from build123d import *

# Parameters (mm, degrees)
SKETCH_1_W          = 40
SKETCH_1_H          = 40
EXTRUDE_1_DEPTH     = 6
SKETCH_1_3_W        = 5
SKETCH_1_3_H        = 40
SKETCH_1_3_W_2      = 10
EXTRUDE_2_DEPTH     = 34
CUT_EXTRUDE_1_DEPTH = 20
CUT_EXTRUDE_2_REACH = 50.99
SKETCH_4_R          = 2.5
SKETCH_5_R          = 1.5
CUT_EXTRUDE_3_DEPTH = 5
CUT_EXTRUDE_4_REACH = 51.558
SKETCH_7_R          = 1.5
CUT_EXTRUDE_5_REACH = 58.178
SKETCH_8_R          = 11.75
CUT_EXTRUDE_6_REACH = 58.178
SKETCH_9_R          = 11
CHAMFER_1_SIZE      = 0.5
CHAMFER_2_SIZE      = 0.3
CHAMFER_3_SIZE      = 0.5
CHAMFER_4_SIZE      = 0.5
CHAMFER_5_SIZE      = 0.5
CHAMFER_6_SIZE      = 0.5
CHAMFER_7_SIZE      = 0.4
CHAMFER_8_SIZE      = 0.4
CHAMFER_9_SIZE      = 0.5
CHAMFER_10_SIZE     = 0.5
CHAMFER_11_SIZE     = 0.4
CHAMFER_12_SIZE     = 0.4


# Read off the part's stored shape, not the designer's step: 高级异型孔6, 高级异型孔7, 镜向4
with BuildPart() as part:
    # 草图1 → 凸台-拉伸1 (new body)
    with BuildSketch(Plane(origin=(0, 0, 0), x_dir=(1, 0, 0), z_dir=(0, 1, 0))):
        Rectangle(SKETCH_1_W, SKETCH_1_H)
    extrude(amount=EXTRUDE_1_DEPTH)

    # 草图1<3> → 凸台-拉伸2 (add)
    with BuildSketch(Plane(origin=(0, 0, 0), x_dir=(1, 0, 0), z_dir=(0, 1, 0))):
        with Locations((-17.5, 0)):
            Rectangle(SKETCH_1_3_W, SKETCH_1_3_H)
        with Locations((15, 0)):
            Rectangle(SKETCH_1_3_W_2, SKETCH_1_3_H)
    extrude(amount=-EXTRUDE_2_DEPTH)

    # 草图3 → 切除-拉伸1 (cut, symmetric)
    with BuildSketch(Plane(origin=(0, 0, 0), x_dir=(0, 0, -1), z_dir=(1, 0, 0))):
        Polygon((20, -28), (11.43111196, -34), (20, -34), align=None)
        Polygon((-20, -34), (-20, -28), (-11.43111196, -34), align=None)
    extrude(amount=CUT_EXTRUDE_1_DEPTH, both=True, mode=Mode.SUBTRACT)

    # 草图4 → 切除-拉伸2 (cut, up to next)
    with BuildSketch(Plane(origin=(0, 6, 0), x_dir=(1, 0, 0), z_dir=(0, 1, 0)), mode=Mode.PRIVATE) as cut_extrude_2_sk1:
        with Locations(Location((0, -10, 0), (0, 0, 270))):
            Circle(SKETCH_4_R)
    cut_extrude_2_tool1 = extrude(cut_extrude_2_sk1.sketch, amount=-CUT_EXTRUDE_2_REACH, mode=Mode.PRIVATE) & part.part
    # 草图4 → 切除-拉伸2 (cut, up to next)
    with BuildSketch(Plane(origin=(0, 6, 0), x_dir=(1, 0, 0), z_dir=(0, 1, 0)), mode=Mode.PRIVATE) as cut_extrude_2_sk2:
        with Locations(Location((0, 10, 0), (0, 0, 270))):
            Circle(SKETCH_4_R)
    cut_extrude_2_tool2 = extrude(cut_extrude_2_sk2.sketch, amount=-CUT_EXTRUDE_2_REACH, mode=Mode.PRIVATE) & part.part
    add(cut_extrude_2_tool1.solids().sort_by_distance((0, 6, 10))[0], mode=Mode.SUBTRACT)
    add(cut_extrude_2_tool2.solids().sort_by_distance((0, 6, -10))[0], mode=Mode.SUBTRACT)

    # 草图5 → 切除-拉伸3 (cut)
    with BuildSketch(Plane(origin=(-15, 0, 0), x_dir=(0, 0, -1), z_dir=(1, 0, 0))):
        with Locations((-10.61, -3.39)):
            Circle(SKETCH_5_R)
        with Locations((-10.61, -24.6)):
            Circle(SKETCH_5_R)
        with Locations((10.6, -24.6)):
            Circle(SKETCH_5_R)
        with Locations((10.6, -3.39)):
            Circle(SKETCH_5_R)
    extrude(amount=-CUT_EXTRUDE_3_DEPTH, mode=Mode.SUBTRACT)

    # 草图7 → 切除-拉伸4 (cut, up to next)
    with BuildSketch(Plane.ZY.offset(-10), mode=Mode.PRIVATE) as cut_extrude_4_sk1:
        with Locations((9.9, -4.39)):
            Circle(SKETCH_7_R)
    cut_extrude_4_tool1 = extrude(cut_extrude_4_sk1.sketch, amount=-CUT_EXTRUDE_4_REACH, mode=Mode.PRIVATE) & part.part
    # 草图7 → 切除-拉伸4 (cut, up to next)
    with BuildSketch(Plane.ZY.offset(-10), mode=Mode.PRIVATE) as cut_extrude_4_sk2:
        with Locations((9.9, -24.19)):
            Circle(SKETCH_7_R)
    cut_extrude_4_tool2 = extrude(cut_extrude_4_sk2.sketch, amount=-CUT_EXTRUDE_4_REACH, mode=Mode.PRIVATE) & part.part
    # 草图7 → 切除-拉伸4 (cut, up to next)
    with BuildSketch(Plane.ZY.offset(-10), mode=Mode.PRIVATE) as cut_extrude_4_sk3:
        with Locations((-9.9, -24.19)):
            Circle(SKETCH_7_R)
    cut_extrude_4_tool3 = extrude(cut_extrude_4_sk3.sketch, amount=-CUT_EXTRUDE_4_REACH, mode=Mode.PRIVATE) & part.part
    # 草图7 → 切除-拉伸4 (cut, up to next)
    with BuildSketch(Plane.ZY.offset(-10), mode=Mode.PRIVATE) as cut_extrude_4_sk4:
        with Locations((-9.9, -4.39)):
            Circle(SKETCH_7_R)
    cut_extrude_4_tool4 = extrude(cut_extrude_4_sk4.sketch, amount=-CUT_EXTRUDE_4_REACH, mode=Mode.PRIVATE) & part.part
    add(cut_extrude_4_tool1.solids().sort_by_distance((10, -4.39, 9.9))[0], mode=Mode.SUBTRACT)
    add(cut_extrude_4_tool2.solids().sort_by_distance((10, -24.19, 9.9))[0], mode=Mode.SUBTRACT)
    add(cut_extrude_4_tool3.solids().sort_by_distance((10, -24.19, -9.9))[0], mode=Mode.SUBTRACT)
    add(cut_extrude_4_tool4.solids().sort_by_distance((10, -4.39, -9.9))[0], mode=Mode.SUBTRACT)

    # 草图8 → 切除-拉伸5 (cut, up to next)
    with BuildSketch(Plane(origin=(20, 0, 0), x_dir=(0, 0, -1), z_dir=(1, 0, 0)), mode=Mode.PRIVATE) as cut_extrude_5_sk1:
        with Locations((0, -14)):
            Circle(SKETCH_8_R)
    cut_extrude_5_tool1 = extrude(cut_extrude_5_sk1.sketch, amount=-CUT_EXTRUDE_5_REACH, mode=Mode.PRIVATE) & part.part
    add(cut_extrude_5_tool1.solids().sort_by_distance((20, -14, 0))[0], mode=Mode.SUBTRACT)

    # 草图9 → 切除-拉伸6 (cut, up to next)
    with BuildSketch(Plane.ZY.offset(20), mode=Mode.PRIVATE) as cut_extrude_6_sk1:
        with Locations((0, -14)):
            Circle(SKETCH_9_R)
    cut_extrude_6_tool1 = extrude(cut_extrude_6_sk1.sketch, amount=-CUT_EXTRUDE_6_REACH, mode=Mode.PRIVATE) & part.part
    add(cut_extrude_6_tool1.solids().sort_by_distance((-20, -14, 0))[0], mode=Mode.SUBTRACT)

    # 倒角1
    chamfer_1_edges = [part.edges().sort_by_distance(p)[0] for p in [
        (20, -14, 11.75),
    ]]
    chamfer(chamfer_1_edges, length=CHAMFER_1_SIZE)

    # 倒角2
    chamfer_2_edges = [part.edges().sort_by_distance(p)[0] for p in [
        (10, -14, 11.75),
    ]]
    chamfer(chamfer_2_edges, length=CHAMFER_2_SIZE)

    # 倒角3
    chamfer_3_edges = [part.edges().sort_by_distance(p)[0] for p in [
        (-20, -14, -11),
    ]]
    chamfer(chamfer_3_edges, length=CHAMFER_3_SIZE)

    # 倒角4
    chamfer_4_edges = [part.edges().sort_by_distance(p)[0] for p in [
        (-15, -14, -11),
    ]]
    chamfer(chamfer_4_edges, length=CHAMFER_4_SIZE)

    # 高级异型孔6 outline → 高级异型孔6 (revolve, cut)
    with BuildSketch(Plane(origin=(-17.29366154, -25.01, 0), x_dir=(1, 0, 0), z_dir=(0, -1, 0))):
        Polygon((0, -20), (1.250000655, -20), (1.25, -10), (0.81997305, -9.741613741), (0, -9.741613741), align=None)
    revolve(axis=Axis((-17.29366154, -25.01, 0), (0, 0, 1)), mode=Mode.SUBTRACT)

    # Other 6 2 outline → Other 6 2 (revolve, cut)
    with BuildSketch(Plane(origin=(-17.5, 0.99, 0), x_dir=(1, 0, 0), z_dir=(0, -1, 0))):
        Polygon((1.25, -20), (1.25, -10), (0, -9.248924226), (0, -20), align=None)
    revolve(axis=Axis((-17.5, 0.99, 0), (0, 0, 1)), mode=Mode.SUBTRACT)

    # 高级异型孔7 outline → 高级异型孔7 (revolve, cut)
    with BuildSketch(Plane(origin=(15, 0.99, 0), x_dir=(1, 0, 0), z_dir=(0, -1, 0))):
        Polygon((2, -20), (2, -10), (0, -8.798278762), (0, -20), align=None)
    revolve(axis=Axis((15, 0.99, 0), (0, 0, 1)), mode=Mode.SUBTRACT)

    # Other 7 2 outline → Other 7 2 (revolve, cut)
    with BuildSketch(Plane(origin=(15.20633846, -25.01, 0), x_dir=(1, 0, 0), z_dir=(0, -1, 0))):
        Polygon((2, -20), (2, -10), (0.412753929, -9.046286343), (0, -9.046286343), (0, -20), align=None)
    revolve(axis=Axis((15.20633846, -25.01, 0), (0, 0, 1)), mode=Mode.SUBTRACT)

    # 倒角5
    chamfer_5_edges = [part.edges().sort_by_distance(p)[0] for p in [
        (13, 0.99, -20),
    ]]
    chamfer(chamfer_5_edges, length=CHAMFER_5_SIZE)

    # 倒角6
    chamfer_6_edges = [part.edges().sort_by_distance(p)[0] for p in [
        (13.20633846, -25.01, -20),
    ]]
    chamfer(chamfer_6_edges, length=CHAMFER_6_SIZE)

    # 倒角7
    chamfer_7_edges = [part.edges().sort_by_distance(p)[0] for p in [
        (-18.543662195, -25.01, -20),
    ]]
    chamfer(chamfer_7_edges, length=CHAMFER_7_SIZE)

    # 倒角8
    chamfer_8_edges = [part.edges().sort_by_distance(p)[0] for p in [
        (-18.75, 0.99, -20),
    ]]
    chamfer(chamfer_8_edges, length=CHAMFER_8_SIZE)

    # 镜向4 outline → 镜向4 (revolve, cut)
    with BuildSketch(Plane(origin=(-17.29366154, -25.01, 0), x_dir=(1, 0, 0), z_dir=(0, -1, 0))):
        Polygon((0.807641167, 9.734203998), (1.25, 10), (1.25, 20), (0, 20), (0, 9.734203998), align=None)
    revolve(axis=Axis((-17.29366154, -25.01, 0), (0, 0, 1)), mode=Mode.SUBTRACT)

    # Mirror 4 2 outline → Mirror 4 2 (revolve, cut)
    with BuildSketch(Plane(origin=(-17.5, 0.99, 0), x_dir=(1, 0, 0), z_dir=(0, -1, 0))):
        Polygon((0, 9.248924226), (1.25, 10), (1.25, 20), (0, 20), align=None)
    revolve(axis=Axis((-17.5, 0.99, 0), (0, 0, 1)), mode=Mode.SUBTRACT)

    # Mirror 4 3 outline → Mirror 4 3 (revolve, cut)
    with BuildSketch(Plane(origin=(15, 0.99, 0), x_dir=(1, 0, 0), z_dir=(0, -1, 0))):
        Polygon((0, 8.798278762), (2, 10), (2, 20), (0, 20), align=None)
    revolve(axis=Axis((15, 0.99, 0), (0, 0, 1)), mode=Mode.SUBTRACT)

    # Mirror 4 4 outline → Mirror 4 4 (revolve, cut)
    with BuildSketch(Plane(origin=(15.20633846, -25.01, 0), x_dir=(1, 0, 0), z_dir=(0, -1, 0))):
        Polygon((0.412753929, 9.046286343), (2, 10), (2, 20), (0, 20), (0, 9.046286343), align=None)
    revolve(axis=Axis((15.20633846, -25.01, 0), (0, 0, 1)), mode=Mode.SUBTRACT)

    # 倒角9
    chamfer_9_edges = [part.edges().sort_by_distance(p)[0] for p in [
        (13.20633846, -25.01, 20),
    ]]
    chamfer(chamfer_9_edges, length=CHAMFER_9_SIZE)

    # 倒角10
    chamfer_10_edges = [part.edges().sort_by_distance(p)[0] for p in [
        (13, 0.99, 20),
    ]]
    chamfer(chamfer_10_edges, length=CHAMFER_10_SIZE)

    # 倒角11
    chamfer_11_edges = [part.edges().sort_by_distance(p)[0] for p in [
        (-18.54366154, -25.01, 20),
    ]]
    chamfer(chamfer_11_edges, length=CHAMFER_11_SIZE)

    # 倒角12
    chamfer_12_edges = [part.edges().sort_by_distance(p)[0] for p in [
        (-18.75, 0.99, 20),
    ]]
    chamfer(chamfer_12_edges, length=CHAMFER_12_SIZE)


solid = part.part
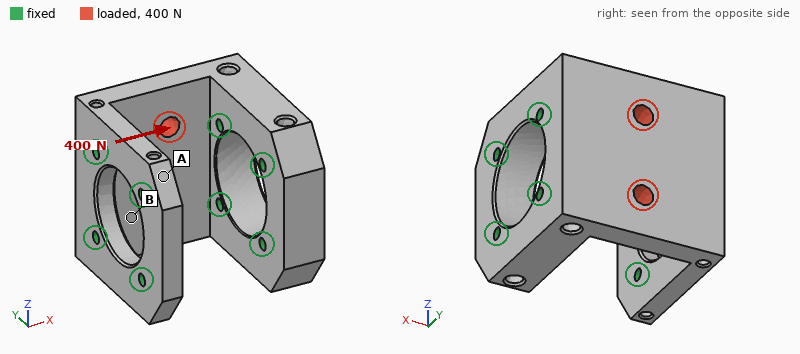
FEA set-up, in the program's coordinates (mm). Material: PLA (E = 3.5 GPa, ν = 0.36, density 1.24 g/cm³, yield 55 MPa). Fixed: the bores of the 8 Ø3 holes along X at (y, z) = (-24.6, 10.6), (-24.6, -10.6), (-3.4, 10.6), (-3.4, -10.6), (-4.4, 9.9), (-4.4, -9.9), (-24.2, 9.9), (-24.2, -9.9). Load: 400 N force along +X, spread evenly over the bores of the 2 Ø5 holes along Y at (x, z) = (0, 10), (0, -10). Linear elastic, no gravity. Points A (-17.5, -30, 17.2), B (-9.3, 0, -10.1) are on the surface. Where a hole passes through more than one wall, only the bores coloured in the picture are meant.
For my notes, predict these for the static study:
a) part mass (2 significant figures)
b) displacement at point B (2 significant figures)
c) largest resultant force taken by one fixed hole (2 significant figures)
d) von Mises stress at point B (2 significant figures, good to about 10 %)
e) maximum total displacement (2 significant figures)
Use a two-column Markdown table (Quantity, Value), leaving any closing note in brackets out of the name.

| Quantity | Value |
|---|---|
| part mass | 27 g |
| displacement at point B | 12 µm |
| largest resultant force taken by one fixed hole | 130 N |
| von Mises stress at point B | 2.2 MPa |
| maximum total displacement | 17 µm |
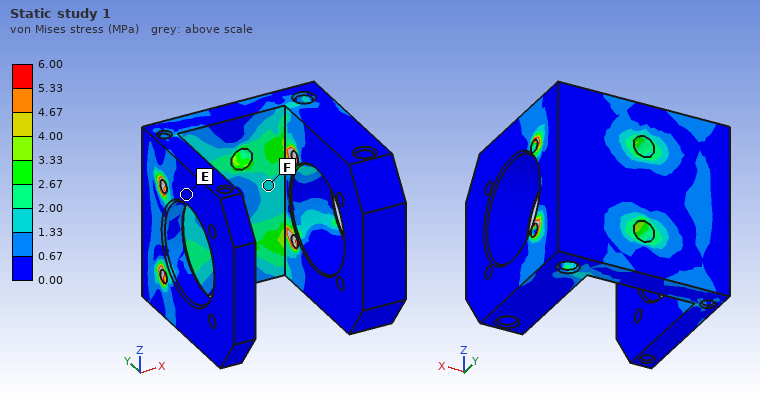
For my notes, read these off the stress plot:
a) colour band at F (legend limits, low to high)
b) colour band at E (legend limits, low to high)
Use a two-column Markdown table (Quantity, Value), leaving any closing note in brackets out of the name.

| Quantity | Value |
|---|---|
| colour band at F | 1.33 to 2.00 MPa |
| colour band at E | 0.00 to 0.67 MPa |
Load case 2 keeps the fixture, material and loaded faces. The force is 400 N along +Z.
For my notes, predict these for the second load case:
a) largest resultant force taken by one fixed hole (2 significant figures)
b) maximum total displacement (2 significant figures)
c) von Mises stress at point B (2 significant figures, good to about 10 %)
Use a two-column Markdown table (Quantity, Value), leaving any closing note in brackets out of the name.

| Quantity | Value |
|---|---|
| largest resultant force taken by one fixed hole | 130 N |
| maximum total displacement | 19 µm |
| von Mises stress at point B | 1.4 MPa |
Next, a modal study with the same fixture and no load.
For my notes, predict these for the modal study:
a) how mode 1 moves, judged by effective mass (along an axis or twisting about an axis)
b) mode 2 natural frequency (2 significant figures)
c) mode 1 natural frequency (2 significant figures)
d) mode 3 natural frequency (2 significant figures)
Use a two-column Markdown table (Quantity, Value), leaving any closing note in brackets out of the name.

| Quantity | Value |
|---|---|
| how mode 1 moves, judged by effective mass | along Y |
| mode 2 natural frequency | 8400 Hz |
| mode 1 natural frequency | 7700 Hz |
| mode 3 natural frequency | 8600 Hz |
